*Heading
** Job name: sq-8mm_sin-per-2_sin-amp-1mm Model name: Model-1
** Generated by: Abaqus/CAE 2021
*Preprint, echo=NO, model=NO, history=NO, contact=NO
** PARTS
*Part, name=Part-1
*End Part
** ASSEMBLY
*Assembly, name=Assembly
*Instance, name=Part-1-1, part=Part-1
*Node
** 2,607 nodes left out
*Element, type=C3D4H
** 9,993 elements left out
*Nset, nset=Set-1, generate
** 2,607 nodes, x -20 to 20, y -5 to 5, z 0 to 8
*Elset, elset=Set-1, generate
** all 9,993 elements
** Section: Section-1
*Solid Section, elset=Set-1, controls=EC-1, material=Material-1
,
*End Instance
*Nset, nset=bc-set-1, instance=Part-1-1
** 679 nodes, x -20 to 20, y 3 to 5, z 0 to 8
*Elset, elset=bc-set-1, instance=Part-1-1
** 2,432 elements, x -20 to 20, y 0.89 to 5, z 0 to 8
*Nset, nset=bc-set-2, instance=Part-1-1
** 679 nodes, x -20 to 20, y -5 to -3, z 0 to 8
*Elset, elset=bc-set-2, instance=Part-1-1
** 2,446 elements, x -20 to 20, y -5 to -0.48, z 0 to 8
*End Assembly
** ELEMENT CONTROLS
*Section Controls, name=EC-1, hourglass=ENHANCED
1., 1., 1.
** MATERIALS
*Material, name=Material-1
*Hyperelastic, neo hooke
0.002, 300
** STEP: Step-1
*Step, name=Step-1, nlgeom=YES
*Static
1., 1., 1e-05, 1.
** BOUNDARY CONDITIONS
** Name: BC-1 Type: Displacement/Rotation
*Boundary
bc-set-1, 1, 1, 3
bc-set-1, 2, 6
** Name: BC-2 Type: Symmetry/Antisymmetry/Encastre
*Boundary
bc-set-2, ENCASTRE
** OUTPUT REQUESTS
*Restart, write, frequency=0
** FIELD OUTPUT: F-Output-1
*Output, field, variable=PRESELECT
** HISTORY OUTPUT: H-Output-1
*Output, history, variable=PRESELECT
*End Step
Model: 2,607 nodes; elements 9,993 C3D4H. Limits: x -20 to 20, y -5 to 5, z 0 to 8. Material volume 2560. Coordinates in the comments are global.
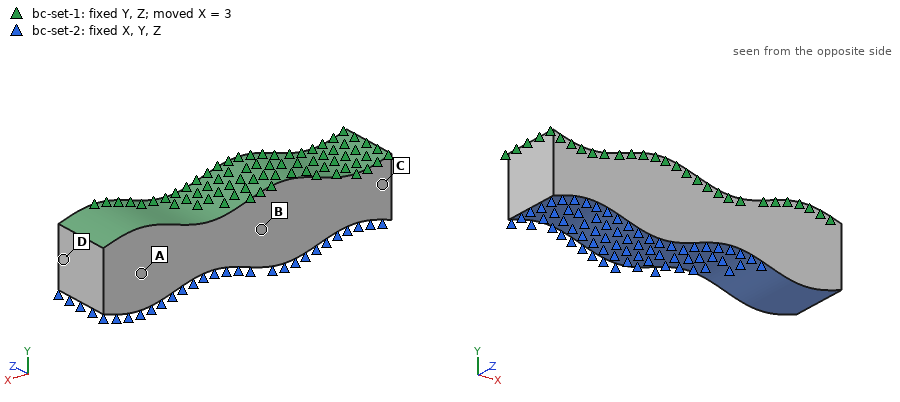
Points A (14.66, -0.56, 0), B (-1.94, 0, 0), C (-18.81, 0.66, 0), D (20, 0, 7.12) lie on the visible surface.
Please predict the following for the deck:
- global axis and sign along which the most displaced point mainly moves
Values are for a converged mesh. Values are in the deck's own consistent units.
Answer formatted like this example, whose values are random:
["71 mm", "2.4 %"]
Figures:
["+X"]
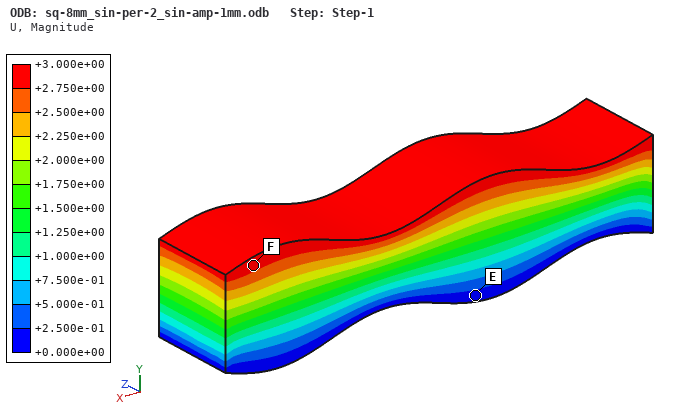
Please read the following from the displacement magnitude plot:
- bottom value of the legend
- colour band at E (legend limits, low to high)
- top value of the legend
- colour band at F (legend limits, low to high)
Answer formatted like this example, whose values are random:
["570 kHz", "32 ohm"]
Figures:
["+0.000e+00", "+0.000e+00 to +2.500e-01", "+3.000e+00", "+2.750e+00 to +3.000e+00"]
